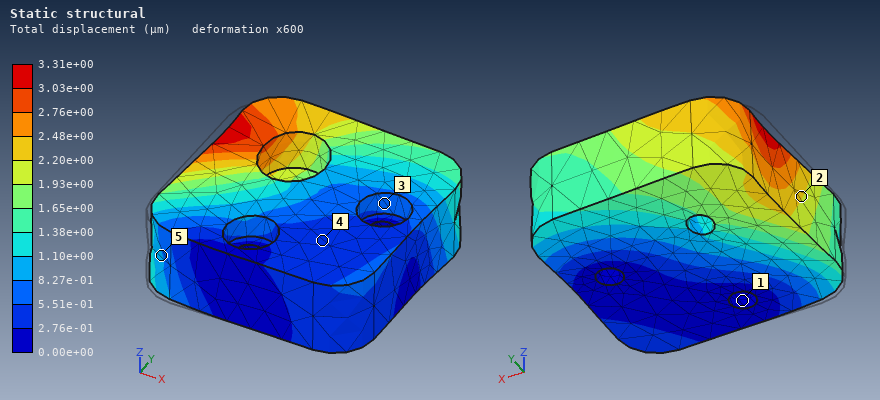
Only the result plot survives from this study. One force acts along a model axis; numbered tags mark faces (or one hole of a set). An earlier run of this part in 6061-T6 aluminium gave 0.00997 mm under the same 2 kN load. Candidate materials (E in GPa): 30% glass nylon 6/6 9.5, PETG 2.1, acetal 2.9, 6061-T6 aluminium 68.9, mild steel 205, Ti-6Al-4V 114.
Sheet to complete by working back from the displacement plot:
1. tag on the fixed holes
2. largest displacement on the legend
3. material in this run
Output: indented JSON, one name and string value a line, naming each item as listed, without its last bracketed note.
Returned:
{
  "tag on the fixed holes": "1",
  "largest displacement on the legend": "3.31e+00 µm",
  "material in this run": "mild steel"
}
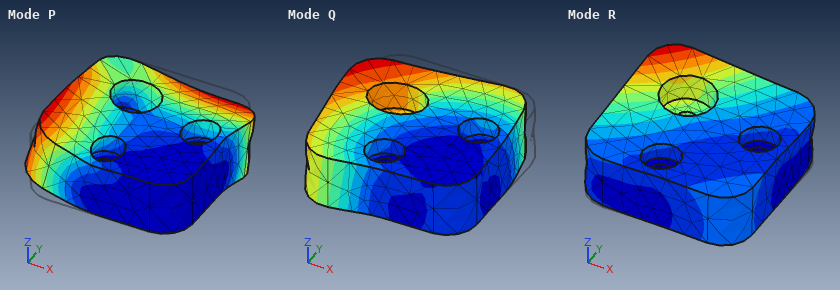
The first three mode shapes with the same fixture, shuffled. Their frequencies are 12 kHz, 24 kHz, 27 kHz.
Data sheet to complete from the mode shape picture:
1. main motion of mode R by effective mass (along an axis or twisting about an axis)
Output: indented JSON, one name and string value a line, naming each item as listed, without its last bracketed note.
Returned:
{
  "main motion of mode R by effective mass": "along Z"
}
